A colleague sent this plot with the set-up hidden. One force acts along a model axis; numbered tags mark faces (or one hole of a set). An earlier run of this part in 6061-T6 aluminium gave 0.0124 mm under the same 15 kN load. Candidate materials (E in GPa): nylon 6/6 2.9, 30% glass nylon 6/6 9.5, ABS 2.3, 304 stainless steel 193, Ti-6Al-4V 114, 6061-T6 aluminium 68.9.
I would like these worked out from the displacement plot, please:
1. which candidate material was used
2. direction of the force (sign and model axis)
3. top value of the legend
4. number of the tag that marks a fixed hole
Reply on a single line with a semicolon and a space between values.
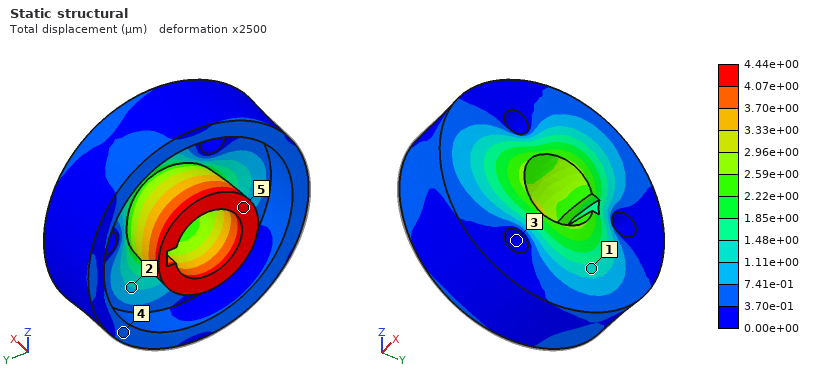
304 stainless steel; +X; 4.44e+00 µm; 3
